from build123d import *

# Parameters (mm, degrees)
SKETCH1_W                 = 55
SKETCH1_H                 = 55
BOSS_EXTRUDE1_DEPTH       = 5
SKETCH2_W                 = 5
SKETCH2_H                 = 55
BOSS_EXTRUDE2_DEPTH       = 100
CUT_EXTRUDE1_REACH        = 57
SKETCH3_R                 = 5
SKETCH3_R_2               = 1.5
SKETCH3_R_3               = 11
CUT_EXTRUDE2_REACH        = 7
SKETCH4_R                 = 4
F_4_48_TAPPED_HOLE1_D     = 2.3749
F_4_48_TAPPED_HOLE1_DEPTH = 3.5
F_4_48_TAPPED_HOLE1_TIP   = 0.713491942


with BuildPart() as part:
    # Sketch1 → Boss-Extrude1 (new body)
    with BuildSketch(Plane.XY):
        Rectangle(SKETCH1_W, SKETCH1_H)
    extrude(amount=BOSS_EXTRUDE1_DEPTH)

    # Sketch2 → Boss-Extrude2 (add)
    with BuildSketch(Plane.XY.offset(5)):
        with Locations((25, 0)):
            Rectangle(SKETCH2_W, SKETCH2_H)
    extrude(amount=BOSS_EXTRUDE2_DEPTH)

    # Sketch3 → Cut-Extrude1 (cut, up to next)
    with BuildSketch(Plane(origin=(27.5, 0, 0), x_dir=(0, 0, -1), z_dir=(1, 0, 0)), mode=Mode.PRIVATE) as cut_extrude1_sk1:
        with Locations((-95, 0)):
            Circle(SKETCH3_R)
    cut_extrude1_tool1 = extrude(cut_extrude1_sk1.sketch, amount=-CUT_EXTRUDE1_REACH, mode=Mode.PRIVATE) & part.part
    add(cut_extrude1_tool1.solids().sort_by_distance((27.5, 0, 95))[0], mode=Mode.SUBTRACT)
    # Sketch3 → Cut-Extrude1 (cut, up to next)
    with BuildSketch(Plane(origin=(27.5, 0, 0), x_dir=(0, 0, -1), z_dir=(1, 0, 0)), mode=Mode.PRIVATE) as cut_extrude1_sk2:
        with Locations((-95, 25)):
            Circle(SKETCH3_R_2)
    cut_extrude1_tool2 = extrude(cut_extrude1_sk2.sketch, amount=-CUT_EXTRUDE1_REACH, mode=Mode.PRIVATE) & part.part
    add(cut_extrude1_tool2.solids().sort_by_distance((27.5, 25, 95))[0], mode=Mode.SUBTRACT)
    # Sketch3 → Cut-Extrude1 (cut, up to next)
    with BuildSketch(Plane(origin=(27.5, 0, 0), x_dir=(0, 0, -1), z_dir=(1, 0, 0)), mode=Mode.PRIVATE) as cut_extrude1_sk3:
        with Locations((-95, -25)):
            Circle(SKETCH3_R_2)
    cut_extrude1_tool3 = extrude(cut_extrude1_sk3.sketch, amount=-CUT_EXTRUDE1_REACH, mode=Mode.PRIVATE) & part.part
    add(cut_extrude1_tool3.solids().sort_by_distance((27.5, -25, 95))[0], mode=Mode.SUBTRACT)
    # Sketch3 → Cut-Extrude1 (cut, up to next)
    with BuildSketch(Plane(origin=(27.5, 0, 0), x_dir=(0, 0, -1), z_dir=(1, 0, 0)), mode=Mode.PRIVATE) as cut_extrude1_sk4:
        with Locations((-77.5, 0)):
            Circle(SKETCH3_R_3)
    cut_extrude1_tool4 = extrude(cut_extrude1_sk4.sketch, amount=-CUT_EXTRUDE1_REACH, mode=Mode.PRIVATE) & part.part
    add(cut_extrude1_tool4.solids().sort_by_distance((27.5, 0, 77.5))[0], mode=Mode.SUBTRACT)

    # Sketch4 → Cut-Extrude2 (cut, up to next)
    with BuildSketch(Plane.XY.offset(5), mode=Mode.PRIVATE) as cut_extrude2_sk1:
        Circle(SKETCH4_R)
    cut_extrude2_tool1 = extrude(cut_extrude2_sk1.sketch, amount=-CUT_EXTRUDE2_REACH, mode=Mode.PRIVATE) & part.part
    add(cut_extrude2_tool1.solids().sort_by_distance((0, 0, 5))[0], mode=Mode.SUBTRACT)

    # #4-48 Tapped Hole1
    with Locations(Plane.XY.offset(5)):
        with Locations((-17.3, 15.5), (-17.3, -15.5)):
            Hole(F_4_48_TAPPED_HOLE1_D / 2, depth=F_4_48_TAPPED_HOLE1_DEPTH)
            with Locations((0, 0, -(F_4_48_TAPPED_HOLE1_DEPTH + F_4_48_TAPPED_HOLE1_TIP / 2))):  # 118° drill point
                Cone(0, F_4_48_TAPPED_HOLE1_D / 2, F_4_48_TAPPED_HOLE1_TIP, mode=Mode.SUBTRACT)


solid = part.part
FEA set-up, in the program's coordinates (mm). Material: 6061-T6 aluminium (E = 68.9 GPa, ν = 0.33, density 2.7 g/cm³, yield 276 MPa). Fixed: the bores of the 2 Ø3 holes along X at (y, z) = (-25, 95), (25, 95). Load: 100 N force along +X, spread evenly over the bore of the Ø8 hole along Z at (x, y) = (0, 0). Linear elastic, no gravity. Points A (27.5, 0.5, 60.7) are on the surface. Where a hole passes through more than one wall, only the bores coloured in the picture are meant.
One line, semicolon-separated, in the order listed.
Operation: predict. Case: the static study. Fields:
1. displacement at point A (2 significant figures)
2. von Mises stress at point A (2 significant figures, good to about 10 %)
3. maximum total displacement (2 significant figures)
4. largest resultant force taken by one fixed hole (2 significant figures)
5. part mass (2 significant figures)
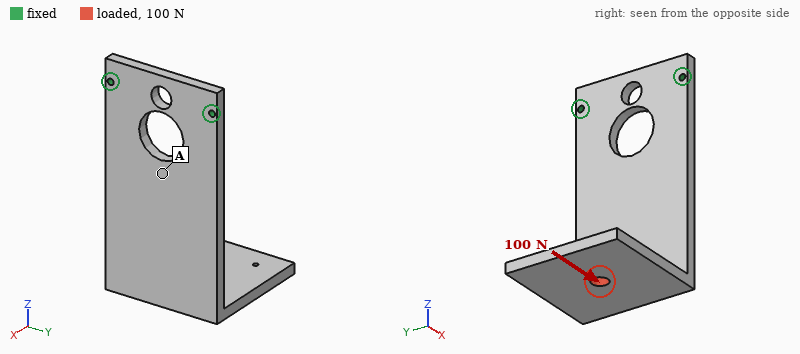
0.23 mm; 14 MPa; 1.3 mm; 50 N; 110 g
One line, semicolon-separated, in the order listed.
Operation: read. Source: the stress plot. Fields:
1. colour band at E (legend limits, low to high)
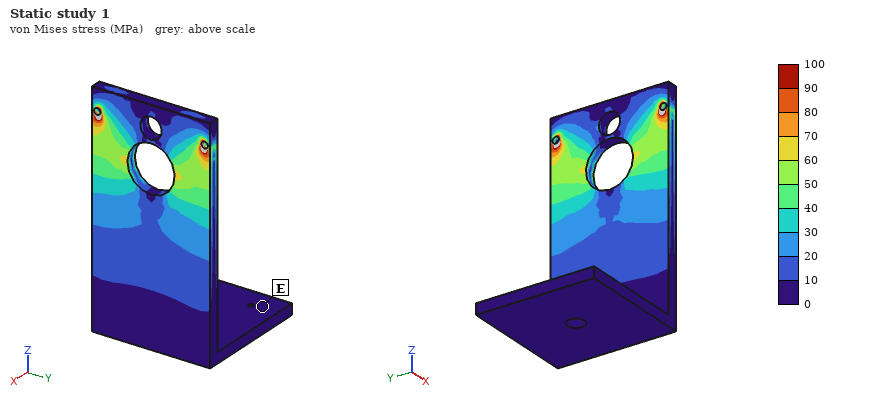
0 to 10 MPa
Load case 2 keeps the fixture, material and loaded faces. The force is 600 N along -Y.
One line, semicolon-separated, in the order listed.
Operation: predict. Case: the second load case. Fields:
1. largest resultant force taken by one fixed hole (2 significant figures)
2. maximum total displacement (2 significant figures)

1.2 kN; 1.3 mm
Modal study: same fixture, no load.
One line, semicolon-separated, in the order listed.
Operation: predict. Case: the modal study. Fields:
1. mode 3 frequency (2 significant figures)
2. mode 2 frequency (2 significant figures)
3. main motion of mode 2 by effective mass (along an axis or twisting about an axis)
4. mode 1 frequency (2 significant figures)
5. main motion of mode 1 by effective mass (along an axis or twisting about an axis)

890 Hz; 590 Hz; along Y; 200 Hz; along X
